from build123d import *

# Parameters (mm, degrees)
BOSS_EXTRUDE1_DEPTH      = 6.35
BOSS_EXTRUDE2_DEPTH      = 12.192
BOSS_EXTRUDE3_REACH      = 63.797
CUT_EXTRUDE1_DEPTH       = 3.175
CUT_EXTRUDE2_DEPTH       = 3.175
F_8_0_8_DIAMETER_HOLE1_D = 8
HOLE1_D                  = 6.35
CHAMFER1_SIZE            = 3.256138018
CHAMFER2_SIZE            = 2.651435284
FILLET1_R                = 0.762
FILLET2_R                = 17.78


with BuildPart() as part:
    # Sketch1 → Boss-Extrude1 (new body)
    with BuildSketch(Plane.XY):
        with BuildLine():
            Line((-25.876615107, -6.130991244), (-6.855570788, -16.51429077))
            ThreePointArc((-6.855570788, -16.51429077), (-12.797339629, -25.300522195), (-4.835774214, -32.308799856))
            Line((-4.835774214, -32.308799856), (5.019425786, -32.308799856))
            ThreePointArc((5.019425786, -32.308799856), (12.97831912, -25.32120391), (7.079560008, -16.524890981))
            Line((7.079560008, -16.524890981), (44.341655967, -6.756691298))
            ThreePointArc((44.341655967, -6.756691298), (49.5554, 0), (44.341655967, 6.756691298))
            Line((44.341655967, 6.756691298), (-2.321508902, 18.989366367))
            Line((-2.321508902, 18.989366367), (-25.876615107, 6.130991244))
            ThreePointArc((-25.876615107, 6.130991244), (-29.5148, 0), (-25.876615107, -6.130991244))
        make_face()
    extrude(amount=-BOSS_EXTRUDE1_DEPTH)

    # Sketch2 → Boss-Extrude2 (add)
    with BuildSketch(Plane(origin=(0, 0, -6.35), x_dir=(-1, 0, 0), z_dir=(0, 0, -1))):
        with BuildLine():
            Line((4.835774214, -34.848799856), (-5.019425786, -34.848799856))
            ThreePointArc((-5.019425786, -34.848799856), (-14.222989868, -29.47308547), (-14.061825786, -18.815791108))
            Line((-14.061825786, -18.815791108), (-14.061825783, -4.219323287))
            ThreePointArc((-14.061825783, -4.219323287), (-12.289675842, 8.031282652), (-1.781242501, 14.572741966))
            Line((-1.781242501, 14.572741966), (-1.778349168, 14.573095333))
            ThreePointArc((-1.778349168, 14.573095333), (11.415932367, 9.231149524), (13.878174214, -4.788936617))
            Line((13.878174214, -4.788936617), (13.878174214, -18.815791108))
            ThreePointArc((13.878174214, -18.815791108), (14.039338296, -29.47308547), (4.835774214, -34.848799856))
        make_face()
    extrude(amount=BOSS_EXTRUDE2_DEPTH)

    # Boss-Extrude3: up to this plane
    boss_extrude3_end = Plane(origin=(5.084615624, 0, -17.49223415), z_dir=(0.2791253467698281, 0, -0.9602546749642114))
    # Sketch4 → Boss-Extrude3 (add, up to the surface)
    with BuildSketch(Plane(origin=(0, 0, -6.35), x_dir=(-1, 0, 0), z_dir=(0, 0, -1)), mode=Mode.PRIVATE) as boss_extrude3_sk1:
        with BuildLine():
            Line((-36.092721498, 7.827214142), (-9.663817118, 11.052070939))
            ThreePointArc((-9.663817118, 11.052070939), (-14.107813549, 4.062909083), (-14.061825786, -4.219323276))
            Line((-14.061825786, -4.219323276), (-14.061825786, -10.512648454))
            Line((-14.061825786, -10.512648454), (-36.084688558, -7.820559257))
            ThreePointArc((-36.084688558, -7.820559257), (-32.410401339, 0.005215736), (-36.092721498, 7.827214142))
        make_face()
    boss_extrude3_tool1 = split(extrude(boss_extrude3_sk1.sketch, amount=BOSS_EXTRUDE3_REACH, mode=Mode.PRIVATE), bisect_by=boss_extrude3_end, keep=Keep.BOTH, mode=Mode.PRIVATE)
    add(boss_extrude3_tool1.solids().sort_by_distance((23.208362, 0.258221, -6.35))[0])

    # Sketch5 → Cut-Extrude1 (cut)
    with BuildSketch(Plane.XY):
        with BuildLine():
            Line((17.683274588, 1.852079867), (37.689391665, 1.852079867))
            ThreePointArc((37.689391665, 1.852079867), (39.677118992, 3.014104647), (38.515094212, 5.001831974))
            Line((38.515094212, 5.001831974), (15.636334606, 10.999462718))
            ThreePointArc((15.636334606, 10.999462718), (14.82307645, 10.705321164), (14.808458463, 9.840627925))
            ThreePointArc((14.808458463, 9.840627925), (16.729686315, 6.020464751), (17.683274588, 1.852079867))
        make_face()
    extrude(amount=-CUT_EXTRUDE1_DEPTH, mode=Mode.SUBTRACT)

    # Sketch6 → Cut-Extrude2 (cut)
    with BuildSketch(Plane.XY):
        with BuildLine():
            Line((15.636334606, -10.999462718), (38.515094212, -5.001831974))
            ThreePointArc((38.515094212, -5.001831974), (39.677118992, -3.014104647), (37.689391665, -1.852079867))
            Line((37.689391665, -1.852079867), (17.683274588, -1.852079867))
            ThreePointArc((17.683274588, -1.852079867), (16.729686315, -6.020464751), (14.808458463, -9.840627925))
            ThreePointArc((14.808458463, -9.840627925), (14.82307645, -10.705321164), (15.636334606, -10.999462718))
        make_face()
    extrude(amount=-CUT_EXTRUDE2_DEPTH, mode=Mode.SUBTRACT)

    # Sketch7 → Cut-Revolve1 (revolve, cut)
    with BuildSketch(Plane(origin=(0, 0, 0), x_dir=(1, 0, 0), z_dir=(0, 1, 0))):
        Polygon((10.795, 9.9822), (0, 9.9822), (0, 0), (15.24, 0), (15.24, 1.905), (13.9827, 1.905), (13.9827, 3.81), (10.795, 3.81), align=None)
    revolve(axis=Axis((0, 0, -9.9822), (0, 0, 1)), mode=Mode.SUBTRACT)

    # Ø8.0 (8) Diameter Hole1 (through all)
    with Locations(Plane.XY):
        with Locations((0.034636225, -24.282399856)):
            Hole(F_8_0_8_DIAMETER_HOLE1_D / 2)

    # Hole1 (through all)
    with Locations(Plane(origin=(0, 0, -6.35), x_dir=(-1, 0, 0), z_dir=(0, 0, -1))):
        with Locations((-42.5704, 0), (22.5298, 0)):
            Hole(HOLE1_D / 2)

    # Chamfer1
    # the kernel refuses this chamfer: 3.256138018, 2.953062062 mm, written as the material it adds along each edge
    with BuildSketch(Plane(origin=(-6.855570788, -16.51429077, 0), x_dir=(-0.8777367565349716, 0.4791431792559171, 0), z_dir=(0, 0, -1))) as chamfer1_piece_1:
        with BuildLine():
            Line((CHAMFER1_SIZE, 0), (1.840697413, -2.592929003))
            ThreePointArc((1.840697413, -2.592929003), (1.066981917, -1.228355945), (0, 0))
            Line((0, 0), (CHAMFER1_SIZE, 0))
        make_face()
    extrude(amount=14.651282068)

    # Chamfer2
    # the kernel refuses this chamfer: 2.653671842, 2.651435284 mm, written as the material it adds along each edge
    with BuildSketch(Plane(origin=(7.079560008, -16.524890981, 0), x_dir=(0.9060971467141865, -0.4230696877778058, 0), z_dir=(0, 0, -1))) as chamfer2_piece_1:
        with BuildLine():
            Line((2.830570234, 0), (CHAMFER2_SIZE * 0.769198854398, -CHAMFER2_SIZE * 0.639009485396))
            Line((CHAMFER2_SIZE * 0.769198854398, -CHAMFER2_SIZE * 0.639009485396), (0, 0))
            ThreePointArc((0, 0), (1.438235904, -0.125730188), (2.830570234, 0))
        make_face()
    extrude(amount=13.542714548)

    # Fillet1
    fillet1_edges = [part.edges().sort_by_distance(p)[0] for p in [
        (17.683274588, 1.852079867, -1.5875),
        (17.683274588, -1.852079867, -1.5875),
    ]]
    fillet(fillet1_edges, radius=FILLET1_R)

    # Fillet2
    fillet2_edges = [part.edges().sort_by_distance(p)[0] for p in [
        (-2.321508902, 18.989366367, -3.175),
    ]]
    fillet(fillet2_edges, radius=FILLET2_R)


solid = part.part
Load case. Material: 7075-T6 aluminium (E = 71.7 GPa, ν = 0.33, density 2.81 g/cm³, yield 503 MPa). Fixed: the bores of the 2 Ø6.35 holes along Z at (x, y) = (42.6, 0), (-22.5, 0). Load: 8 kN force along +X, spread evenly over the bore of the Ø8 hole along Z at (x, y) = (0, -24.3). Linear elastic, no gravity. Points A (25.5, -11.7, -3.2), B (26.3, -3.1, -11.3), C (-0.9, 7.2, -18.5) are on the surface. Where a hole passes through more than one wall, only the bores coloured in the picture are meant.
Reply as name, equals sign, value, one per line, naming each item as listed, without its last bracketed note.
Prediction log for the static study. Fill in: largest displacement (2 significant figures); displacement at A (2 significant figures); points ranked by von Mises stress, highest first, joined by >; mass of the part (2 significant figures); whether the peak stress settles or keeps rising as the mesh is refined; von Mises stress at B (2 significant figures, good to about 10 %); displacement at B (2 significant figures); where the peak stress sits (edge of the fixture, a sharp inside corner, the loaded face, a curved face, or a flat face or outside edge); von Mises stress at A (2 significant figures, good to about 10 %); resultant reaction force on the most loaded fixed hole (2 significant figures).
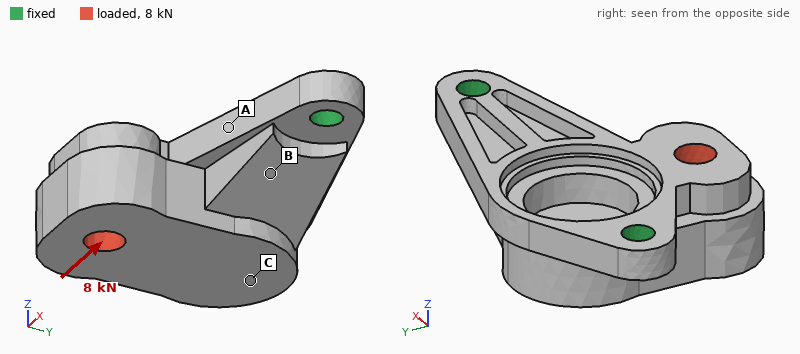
largest displacement = 0.11 mm
displacement at A = 0.036 mm
points ranked by von Mises stress, highest first, joined by > = A > B > C
mass of the part = 71 g
whether the peak stress settles or keeps rising as the mesh is refined = keeps rising
von Mises stress at B = 39 MPa
displacement at B = 0.026 mm
where the peak stress sits = a sharp inside corner
von Mises stress at A = 94 MPa
resultant reaction force on the most loaded fixed hole = 5.4 kN
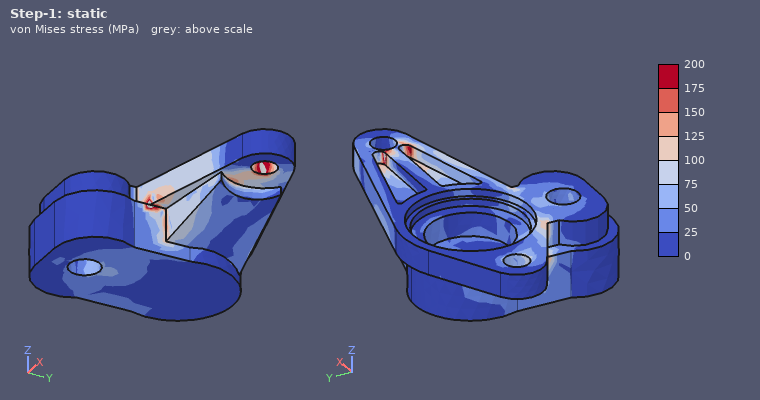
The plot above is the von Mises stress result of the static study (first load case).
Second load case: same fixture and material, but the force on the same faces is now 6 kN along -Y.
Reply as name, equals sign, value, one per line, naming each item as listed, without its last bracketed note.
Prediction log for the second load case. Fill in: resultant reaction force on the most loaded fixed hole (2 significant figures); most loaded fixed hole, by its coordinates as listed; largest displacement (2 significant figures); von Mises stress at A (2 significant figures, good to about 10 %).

resultant reaction force on the most loaded fixed hole = 4.0 kN
most loaded fixed hole, by its coordinates as listed = (-22.5, 0)
largest displacement = 0.20 mm
von Mises stress at A = 42 MPa
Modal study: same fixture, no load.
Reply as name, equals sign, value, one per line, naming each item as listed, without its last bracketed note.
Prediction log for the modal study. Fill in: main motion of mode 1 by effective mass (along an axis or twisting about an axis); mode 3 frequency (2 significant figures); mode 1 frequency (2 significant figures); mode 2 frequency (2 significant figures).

main motion of mode 1 by effective mass = along Z
mode 3 frequency = 9000 Hz
mode 1 frequency = 2600 Hz
mode 2 frequency = 7500 Hz
